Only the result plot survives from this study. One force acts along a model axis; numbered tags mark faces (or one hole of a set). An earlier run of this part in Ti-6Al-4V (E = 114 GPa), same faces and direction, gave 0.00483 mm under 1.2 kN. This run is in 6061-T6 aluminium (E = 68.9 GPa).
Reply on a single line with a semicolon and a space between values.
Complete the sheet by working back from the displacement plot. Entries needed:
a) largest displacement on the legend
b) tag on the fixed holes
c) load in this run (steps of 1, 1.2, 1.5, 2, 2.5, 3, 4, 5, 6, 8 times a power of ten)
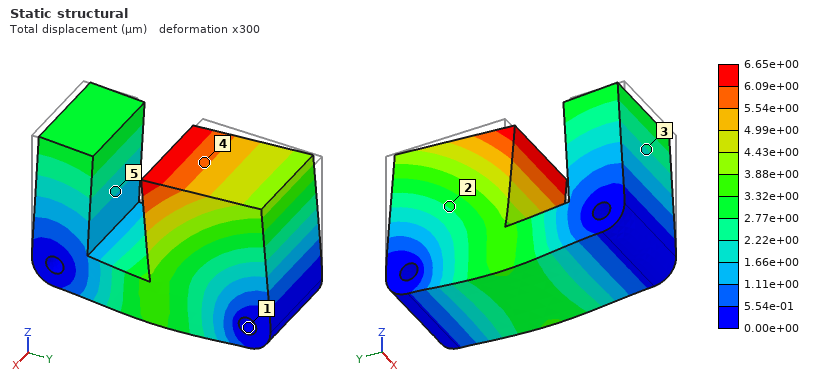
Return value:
6.65e+00 µm; 1; 1 kN
